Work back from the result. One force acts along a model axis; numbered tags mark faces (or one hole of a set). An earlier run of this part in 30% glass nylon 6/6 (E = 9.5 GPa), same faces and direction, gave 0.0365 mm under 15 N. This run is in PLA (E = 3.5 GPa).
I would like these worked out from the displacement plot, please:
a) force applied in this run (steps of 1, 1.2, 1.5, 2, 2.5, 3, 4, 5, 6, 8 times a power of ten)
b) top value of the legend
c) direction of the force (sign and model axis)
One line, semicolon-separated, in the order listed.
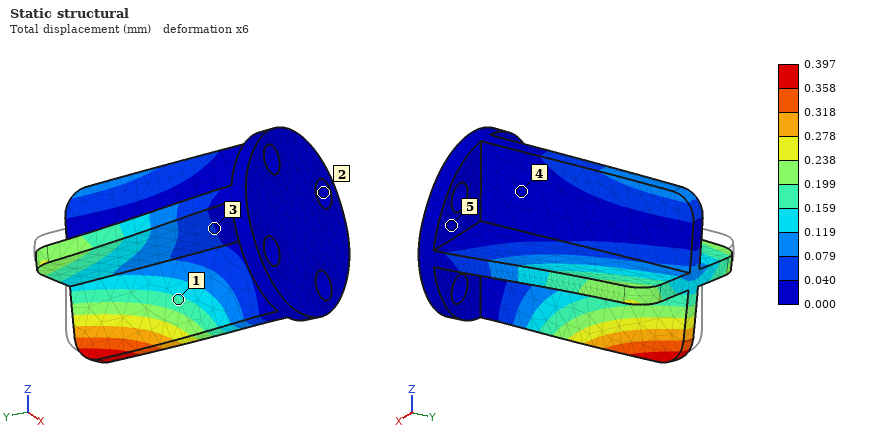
60 N; 0.397 mm; +X
